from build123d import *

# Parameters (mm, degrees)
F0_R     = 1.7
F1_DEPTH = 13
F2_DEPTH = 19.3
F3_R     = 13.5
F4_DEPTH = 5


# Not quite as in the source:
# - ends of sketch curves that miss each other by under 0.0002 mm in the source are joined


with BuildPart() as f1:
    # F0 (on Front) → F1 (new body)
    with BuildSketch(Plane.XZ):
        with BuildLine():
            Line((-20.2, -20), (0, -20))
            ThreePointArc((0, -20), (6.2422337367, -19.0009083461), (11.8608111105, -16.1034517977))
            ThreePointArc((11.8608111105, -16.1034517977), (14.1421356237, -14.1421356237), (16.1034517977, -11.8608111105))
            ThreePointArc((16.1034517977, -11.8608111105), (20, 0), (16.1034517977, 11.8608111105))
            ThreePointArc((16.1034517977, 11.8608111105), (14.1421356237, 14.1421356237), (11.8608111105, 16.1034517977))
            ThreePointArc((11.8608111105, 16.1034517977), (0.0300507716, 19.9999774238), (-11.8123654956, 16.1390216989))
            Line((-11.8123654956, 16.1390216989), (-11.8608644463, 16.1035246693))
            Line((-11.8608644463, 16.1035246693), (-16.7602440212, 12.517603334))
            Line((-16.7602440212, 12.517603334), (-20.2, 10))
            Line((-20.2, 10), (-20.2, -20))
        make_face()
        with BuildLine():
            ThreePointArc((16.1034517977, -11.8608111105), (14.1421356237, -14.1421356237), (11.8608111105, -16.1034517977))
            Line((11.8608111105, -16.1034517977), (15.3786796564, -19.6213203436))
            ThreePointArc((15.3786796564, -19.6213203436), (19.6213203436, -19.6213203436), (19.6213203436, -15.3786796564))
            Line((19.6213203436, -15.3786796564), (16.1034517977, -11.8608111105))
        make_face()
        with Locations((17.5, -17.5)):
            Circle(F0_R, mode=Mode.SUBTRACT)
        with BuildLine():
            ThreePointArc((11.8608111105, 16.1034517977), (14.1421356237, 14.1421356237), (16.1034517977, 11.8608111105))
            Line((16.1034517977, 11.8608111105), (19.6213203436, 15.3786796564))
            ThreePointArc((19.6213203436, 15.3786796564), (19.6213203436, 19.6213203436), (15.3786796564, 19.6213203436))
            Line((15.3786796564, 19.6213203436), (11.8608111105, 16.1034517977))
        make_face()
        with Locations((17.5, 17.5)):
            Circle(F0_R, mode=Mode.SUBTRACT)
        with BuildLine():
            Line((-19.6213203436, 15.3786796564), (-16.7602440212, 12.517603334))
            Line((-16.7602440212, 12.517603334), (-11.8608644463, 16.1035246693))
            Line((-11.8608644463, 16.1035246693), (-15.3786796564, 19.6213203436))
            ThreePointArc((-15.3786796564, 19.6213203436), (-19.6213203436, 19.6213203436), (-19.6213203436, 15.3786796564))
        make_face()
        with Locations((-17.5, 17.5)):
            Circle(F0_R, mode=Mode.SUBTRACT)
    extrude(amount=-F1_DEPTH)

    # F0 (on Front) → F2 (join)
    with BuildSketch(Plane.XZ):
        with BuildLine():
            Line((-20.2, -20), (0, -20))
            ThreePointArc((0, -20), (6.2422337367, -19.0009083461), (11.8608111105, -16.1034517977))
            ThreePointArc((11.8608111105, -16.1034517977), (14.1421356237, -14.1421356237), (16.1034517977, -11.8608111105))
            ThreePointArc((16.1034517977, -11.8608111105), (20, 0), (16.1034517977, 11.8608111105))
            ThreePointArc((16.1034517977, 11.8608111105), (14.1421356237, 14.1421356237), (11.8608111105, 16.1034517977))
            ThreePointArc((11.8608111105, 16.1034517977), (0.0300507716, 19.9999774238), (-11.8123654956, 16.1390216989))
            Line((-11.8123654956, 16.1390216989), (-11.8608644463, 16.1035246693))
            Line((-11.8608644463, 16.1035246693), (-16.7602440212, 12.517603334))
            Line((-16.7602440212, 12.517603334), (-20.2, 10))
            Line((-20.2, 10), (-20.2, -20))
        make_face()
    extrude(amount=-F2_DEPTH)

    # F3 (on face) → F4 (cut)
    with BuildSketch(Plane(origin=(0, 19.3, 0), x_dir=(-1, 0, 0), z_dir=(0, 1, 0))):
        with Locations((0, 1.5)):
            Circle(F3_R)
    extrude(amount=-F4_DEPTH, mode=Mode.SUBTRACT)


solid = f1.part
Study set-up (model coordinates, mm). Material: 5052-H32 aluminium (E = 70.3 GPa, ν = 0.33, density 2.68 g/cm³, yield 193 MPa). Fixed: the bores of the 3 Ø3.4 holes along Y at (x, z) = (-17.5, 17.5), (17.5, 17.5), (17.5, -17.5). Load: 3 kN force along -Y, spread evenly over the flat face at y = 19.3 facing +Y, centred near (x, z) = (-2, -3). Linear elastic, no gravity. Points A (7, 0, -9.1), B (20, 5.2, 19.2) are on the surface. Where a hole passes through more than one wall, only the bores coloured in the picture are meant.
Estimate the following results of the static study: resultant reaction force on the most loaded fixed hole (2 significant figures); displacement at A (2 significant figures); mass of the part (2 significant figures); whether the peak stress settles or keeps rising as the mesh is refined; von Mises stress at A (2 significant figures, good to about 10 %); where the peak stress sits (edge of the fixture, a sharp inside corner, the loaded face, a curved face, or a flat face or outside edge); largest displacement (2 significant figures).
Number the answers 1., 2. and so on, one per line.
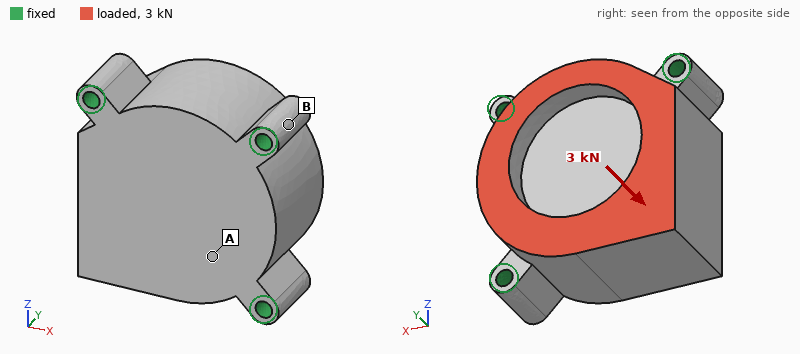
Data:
1. 1.5 kN
2. 10 µm
3. 66 g
4. keeps rising
5. 15 MPa
6. edge of the fixture
7. 37 µm
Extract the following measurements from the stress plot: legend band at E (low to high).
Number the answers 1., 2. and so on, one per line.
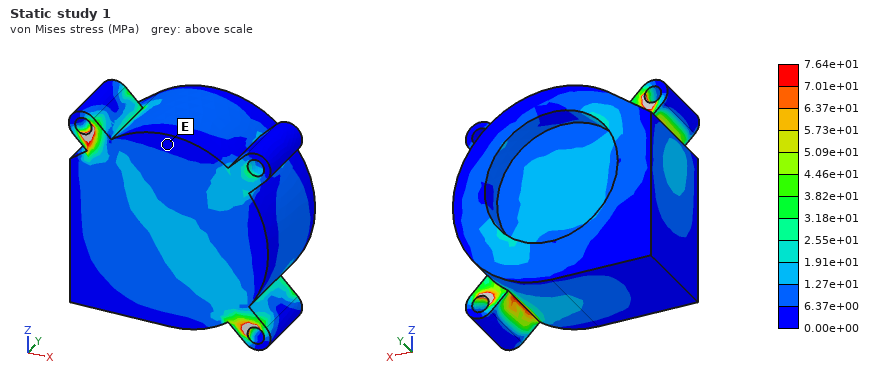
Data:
1. 0.00e+00 to 6.37e+00 MPa
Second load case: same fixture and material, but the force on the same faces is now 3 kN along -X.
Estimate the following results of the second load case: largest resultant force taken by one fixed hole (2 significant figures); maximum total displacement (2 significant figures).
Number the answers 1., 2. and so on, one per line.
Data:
1. 1.5 kN
2. 28 µm
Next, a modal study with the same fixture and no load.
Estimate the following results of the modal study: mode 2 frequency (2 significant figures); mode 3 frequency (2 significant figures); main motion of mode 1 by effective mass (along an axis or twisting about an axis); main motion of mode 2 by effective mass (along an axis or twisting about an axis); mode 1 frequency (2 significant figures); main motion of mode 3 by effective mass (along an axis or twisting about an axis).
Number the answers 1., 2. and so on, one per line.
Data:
1. 19 kHz
2. 20 kHz
3. along Y
4. along X
5. 8200 Hz
6. along Z
